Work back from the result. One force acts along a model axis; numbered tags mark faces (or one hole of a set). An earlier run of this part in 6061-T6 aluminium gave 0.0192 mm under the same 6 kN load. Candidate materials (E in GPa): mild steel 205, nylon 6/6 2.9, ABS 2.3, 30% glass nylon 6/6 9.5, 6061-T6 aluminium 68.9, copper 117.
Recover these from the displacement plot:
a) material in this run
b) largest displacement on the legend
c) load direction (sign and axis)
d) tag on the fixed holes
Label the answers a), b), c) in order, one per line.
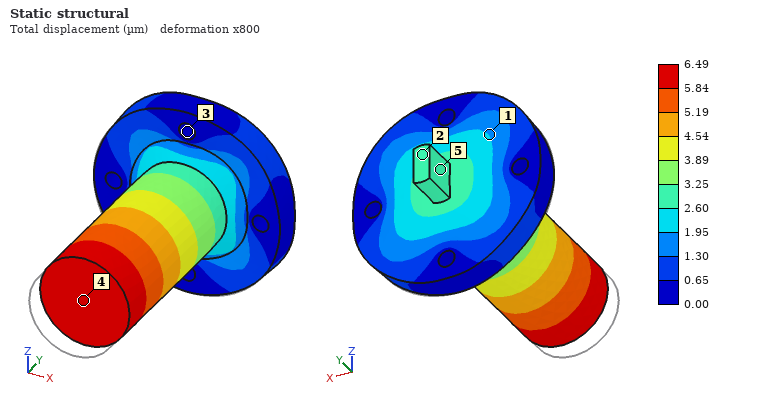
a) mild steel
b) 6.49 µm
c) +Y
d) 3
